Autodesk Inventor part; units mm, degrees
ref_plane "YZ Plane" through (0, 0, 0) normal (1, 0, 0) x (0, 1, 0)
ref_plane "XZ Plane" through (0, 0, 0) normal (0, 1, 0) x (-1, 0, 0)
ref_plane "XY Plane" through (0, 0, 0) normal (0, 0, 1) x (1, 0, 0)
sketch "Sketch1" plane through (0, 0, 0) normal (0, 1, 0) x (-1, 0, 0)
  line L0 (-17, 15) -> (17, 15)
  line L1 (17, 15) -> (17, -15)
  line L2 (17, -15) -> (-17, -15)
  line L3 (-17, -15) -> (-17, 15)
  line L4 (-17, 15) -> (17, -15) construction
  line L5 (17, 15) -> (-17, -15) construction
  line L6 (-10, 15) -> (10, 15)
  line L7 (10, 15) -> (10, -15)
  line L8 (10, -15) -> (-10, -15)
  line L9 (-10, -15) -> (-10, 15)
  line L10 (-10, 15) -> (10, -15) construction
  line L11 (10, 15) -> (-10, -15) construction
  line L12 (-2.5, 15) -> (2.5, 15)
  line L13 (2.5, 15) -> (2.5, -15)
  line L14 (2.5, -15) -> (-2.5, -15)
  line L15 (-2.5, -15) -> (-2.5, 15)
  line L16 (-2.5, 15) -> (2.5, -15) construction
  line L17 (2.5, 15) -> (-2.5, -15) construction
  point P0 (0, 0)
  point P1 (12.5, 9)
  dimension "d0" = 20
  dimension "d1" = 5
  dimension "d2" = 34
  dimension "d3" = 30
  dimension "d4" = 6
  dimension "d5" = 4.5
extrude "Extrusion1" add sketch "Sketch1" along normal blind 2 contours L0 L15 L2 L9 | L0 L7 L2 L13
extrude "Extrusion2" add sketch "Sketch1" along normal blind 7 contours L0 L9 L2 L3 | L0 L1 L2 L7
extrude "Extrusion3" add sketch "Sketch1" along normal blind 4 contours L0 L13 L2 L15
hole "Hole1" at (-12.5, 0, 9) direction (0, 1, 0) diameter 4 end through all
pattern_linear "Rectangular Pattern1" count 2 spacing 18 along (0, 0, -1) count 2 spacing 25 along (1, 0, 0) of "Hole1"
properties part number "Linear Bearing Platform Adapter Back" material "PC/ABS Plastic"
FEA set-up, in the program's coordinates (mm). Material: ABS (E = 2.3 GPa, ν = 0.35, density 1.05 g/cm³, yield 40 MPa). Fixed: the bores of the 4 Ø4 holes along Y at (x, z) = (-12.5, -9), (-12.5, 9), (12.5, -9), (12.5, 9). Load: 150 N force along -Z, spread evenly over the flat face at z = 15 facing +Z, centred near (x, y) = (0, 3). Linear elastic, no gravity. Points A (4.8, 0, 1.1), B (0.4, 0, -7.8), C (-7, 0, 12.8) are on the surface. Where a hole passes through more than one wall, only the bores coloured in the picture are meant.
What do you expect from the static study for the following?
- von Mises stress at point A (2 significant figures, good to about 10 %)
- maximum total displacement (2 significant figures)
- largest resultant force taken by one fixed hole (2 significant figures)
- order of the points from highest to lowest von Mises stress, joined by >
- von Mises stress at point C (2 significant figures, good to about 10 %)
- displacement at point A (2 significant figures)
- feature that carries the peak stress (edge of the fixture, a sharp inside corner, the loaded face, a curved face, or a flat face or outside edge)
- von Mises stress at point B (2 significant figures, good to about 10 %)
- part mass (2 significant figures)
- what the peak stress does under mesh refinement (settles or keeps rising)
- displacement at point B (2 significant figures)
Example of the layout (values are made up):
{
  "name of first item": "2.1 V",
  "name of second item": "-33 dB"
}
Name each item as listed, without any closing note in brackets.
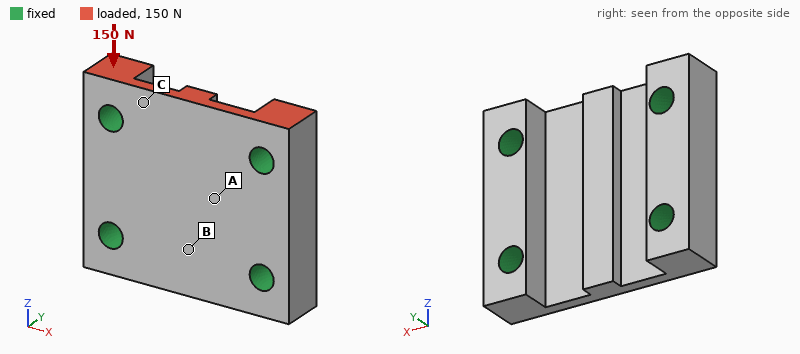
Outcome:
{
  "von Mises stress at point A": "0.58 MPa",
  "maximum total displacement": "11 µm",
  "largest resultant force taken by one fixed hole": "65 N",
  "order of the points from highest to lowest von Mises stress, joined by >": "C > A > B",
  "von Mises stress at point C": "0.90 MPa",
  "displacement at point A": "2.9 µm",
  "feature that carries the peak stress": "edge of the fixture",
  "von Mises stress at point B": "0.21 MPa",
  "part mass": "4.3 g",
  "what the peak stress does under mesh refinement": "keeps rising",
  "displacement at point B": "3.1 µm"
}
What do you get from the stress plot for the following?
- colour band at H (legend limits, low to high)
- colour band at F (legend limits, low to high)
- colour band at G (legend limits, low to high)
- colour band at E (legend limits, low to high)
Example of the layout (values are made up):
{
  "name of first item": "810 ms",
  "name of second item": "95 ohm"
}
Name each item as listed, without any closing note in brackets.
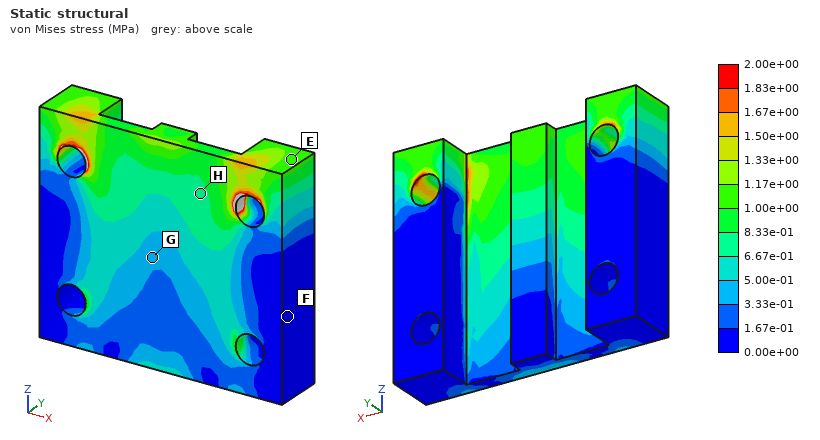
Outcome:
{
  "colour band at H": "6.67e-01 to 8.33e-01 MPa",
  "colour band at F": "0.00e+00 to 1.67e-01 MPa",
  "colour band at G": "3.33e-01 to 5.00e-01 MPa",
  "colour band at E": "1.00e+00 to 1.17e+00 MPa"
}
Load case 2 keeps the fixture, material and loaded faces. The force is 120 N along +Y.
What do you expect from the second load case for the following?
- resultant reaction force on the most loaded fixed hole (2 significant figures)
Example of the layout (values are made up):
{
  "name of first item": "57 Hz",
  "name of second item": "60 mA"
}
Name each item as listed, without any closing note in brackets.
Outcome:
{
  "resultant reaction force on the most loaded fixed hole": "63 N"
}
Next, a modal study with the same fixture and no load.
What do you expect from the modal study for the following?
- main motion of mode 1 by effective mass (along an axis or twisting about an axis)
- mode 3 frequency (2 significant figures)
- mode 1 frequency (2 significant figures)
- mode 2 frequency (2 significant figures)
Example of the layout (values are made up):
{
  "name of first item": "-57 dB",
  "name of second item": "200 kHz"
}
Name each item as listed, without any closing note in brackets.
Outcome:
{
  "main motion of mode 1 by effective mass": "along Y",
  "mode 3 frequency": "9500 Hz",
  "mode 1 frequency": "5800 Hz",
  "mode 2 frequency": "6200 Hz"
}
